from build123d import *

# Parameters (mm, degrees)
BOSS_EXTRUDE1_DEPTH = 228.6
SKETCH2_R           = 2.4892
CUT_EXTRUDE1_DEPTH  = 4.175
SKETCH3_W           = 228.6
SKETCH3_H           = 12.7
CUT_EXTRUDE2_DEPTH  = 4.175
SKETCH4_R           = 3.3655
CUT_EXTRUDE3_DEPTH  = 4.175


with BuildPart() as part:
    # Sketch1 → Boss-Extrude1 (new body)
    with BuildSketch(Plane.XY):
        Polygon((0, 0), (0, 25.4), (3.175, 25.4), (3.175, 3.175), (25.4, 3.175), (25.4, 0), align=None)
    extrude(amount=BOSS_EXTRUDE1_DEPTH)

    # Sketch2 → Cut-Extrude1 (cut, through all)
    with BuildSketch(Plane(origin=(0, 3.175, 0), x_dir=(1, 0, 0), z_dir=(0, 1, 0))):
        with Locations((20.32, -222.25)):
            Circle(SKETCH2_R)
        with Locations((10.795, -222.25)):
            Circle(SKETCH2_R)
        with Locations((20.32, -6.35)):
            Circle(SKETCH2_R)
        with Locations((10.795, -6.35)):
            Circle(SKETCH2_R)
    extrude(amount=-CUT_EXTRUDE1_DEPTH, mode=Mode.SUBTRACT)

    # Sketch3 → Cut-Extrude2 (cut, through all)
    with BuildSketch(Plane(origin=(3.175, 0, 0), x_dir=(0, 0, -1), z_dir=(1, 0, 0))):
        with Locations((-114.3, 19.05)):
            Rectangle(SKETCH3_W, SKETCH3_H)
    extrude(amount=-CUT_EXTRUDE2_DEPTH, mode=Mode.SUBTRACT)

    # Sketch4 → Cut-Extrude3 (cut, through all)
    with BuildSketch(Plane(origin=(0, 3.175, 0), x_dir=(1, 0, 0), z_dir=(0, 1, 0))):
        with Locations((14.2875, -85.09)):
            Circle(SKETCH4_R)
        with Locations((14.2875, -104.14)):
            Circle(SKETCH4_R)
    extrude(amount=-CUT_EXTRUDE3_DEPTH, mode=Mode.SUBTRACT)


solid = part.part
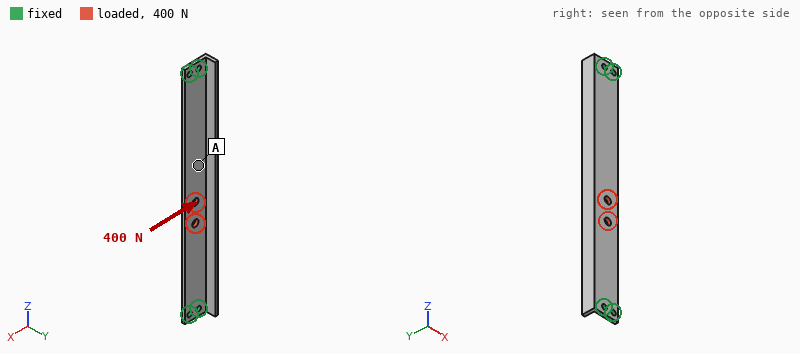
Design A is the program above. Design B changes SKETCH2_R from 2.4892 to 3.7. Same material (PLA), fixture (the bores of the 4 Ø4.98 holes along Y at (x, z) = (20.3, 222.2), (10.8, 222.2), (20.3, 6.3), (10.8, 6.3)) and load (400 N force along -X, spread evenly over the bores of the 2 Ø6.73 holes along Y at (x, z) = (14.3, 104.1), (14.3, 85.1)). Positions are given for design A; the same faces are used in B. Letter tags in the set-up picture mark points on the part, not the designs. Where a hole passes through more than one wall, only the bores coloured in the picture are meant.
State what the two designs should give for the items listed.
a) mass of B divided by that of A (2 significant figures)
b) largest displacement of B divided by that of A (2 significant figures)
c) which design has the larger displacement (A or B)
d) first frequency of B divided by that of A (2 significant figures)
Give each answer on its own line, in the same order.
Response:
0.99
0.91
A
1.1
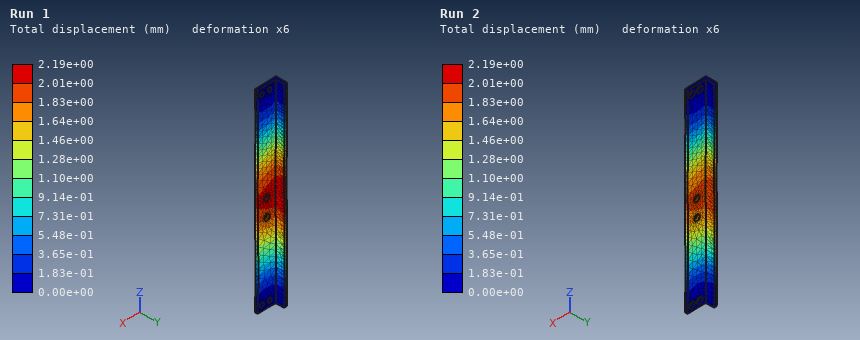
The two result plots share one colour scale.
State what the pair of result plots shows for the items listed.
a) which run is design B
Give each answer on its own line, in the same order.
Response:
Run 2
